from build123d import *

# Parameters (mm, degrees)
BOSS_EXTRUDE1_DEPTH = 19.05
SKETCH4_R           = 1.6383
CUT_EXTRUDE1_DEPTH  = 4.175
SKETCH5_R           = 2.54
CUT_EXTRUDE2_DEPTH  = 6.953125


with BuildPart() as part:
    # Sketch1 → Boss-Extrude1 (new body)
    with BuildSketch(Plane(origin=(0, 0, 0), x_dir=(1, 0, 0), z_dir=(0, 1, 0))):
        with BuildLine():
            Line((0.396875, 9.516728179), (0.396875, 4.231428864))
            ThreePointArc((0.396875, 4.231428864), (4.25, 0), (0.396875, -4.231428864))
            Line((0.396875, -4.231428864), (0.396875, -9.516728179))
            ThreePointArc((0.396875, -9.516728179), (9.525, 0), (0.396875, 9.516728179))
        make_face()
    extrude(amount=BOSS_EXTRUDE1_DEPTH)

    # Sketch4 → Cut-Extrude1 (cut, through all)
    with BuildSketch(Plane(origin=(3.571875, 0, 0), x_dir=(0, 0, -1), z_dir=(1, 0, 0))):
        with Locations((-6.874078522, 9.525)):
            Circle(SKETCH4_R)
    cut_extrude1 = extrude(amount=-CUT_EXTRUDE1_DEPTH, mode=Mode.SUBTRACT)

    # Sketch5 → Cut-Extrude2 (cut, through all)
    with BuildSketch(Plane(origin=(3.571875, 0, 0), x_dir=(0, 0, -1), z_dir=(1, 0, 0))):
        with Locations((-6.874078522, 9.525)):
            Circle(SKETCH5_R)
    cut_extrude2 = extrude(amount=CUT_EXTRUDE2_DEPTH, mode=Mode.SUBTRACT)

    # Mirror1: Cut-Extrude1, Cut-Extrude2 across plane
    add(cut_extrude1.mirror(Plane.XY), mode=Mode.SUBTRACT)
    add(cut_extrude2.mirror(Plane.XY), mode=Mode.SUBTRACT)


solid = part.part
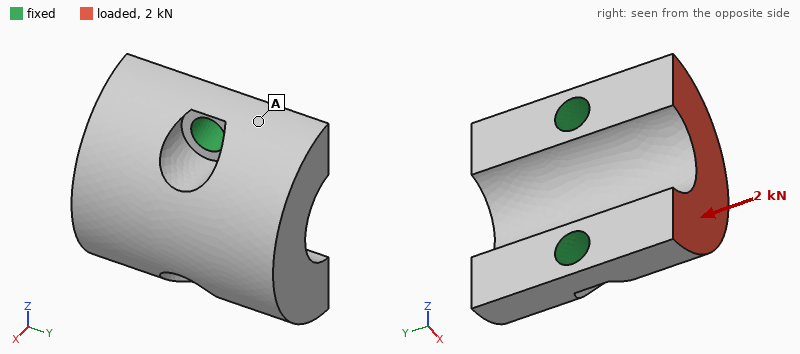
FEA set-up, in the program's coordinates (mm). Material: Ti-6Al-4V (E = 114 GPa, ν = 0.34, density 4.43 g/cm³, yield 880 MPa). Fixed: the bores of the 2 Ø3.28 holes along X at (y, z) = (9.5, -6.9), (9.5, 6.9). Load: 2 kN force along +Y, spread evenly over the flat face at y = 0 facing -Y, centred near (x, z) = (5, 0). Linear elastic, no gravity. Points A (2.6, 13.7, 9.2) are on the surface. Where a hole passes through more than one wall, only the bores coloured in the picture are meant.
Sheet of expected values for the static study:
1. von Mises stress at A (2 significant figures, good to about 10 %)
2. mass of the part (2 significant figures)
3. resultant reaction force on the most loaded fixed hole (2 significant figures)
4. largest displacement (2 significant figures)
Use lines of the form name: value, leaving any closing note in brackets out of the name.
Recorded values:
von Mises stress at A: 28 MPa
mass of the part: 8.5 g
resultant reaction force on the most loaded fixed hole: 1.0 kN
largest displacement: 17 µm
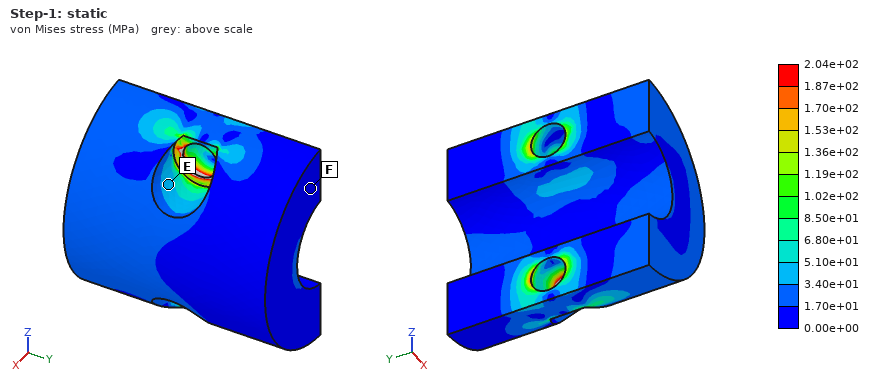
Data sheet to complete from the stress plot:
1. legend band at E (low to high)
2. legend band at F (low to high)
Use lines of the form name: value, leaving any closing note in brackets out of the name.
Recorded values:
legend band at E: 3.40e+01 to 5.10e+01 MPa
legend band at F: 0.00e+00 to 1.70e+01 MPa
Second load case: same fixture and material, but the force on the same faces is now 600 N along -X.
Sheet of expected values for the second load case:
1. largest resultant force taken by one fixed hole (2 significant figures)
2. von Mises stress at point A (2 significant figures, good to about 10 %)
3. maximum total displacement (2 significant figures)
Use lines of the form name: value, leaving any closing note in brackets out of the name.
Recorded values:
largest resultant force taken by one fixed hole: 330 N
von Mises stress at point A: 21 MPa
maximum total displacement: 17 µm
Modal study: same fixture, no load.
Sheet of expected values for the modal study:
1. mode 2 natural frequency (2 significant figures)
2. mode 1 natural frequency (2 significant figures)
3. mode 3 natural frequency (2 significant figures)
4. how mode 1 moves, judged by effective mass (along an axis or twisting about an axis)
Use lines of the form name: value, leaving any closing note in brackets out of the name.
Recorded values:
mode 2 natural frequency: 42 kHz
mode 1 natural frequency: 18 kHz
mode 3 natural frequency: 43 kHz
how mode 1 moves, judged by effective mass: along Y
